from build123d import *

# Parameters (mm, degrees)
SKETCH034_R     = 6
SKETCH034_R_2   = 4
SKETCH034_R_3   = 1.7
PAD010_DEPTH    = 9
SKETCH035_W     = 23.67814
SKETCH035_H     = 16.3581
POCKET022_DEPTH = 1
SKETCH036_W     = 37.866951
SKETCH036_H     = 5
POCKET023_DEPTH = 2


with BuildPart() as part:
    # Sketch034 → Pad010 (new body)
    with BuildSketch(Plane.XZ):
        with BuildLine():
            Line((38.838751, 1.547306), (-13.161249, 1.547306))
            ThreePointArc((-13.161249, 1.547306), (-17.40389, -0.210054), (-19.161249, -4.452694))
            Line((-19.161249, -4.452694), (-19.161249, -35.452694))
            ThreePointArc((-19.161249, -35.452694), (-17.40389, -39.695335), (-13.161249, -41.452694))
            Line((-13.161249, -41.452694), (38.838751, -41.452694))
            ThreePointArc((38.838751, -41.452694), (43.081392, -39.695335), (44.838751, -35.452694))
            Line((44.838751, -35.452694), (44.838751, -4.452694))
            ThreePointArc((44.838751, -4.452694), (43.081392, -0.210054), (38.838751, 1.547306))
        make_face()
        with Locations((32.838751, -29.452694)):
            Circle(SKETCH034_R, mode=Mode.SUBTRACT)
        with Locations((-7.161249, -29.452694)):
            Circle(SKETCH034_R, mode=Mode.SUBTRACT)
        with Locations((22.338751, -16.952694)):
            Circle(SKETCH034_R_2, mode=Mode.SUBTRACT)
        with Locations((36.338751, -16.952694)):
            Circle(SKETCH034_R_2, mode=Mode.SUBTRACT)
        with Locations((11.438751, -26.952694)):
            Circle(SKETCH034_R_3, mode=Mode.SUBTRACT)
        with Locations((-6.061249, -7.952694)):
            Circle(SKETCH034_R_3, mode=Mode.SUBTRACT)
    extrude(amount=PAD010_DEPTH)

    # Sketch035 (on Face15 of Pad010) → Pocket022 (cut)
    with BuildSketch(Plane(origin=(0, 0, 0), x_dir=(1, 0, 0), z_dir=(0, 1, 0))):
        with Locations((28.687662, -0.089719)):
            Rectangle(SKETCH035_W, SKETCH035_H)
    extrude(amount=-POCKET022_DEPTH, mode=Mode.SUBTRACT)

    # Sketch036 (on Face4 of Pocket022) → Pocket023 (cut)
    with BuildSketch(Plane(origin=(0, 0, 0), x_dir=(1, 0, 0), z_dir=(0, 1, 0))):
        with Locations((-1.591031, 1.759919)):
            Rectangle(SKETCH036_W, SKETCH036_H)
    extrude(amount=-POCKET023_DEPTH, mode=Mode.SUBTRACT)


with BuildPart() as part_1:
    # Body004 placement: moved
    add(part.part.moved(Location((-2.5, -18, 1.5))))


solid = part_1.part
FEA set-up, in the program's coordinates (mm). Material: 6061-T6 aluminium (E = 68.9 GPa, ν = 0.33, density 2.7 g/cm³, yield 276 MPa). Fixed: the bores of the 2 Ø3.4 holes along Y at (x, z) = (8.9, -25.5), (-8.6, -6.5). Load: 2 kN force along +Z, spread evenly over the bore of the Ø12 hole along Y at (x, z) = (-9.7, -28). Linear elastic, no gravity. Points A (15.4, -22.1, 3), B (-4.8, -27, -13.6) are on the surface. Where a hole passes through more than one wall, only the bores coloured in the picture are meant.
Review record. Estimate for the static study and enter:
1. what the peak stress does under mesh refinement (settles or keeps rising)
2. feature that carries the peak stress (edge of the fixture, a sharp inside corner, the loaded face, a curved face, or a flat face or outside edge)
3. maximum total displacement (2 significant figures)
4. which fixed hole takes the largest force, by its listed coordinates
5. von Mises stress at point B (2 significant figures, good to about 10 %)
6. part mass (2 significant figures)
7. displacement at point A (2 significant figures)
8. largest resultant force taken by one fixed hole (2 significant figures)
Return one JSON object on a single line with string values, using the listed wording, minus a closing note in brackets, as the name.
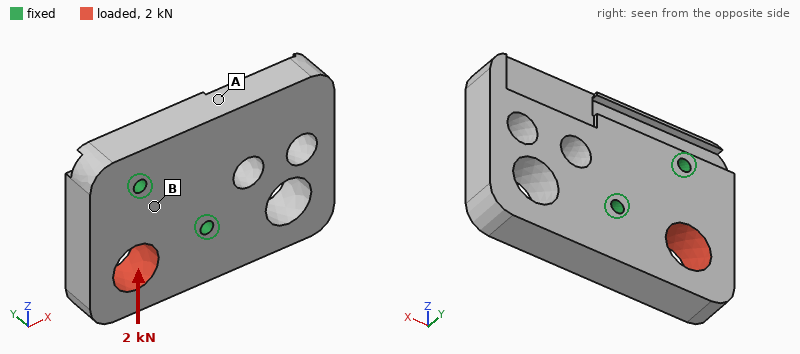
{"what the peak stress does under mesh refinement": "keeps rising", "feature that carries the peak stress": "edge of the fixture", "maximum total displacement": "7.3 µm", "which fixed hole takes the largest force, by its listed coordinates": "(-8.6, -6.5)", "von Mises stress at point B": "8.4 MPa", "part mass": "56 g", "displacement at point A": "1.2 µm", "largest resultant force taken by one fixed hole": "1.6 kN"}
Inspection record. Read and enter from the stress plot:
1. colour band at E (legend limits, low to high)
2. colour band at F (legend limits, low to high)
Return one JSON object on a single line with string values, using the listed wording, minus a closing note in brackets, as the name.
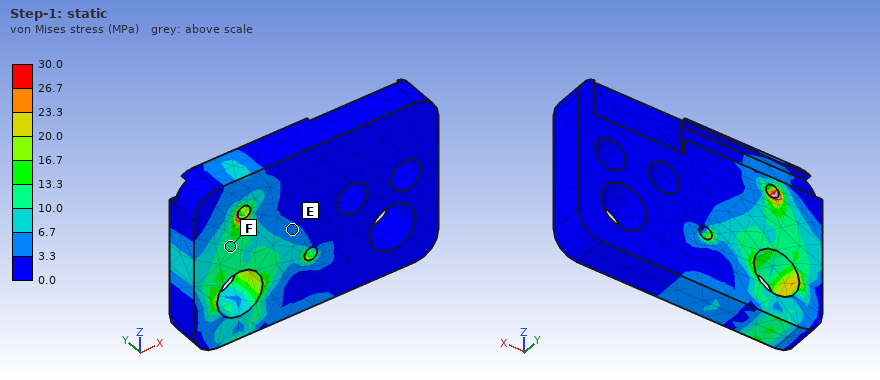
{"colour band at E": "3.3 to 6.7 MPa", "colour band at F": "10.0 to 13.3 MPa"}
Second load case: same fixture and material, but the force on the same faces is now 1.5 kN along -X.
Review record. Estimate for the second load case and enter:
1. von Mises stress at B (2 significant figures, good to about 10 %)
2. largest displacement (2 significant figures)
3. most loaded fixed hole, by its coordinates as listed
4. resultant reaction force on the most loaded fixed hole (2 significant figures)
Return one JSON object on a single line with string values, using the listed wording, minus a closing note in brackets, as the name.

{"von Mises stress at B": "4.7 MPa", "largest displacement": "5.7 µm", "most loaded fixed hole, by its coordinates as listed": "(8.9, -25.5)", "resultant reaction force on the most loaded fixed hole": "1.4 kN"}
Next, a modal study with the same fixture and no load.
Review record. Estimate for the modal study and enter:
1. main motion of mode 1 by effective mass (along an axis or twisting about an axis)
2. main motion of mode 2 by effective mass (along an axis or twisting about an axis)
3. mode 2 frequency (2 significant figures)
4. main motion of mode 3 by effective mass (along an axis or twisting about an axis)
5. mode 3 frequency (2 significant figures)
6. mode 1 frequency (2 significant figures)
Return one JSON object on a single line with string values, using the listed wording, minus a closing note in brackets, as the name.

{"main motion of mode 1 by effective mass": "along Y", "main motion of mode 2 by effective mass": "twisting about X", "mode 2 frequency": "8100 Hz", "main motion of mode 3 by effective mass": "along Y", "mode 3 frequency": "11 kHz", "mode 1 frequency": "4600 Hz"}
